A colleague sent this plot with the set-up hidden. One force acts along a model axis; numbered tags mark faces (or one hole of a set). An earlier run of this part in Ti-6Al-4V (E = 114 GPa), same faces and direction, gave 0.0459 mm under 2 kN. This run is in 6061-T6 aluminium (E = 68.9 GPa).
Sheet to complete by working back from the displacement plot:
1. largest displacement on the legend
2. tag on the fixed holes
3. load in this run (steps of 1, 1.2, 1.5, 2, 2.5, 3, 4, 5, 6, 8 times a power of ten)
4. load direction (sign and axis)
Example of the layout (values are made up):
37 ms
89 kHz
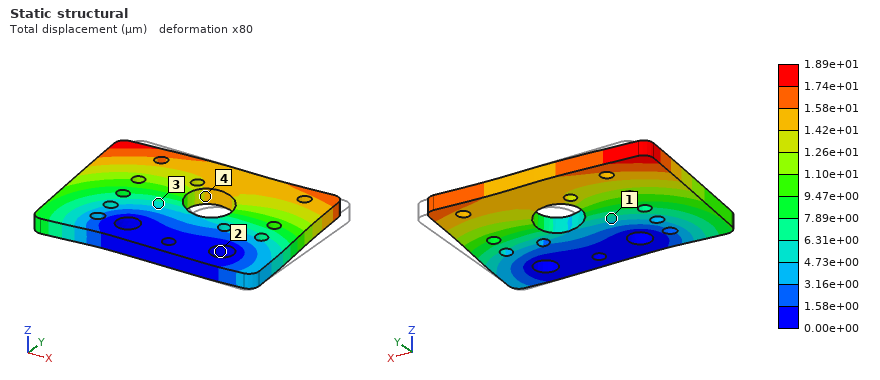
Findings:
1.89e+01 µm
2
500 N
-X
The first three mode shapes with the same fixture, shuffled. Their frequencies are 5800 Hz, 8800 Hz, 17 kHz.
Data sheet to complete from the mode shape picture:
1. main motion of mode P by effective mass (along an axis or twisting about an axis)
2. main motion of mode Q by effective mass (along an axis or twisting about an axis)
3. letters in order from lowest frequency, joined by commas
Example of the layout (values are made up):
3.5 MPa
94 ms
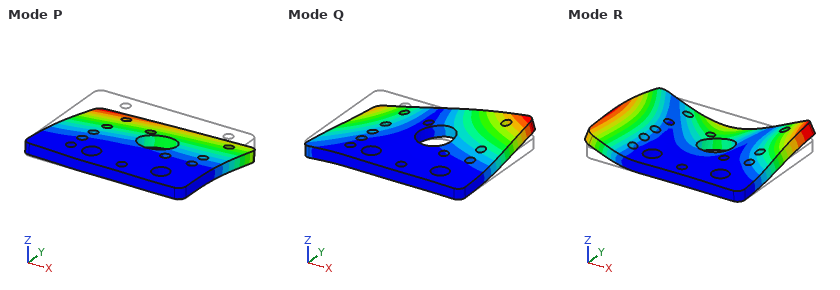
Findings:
along Z
twisting about Y
P, Q, R
